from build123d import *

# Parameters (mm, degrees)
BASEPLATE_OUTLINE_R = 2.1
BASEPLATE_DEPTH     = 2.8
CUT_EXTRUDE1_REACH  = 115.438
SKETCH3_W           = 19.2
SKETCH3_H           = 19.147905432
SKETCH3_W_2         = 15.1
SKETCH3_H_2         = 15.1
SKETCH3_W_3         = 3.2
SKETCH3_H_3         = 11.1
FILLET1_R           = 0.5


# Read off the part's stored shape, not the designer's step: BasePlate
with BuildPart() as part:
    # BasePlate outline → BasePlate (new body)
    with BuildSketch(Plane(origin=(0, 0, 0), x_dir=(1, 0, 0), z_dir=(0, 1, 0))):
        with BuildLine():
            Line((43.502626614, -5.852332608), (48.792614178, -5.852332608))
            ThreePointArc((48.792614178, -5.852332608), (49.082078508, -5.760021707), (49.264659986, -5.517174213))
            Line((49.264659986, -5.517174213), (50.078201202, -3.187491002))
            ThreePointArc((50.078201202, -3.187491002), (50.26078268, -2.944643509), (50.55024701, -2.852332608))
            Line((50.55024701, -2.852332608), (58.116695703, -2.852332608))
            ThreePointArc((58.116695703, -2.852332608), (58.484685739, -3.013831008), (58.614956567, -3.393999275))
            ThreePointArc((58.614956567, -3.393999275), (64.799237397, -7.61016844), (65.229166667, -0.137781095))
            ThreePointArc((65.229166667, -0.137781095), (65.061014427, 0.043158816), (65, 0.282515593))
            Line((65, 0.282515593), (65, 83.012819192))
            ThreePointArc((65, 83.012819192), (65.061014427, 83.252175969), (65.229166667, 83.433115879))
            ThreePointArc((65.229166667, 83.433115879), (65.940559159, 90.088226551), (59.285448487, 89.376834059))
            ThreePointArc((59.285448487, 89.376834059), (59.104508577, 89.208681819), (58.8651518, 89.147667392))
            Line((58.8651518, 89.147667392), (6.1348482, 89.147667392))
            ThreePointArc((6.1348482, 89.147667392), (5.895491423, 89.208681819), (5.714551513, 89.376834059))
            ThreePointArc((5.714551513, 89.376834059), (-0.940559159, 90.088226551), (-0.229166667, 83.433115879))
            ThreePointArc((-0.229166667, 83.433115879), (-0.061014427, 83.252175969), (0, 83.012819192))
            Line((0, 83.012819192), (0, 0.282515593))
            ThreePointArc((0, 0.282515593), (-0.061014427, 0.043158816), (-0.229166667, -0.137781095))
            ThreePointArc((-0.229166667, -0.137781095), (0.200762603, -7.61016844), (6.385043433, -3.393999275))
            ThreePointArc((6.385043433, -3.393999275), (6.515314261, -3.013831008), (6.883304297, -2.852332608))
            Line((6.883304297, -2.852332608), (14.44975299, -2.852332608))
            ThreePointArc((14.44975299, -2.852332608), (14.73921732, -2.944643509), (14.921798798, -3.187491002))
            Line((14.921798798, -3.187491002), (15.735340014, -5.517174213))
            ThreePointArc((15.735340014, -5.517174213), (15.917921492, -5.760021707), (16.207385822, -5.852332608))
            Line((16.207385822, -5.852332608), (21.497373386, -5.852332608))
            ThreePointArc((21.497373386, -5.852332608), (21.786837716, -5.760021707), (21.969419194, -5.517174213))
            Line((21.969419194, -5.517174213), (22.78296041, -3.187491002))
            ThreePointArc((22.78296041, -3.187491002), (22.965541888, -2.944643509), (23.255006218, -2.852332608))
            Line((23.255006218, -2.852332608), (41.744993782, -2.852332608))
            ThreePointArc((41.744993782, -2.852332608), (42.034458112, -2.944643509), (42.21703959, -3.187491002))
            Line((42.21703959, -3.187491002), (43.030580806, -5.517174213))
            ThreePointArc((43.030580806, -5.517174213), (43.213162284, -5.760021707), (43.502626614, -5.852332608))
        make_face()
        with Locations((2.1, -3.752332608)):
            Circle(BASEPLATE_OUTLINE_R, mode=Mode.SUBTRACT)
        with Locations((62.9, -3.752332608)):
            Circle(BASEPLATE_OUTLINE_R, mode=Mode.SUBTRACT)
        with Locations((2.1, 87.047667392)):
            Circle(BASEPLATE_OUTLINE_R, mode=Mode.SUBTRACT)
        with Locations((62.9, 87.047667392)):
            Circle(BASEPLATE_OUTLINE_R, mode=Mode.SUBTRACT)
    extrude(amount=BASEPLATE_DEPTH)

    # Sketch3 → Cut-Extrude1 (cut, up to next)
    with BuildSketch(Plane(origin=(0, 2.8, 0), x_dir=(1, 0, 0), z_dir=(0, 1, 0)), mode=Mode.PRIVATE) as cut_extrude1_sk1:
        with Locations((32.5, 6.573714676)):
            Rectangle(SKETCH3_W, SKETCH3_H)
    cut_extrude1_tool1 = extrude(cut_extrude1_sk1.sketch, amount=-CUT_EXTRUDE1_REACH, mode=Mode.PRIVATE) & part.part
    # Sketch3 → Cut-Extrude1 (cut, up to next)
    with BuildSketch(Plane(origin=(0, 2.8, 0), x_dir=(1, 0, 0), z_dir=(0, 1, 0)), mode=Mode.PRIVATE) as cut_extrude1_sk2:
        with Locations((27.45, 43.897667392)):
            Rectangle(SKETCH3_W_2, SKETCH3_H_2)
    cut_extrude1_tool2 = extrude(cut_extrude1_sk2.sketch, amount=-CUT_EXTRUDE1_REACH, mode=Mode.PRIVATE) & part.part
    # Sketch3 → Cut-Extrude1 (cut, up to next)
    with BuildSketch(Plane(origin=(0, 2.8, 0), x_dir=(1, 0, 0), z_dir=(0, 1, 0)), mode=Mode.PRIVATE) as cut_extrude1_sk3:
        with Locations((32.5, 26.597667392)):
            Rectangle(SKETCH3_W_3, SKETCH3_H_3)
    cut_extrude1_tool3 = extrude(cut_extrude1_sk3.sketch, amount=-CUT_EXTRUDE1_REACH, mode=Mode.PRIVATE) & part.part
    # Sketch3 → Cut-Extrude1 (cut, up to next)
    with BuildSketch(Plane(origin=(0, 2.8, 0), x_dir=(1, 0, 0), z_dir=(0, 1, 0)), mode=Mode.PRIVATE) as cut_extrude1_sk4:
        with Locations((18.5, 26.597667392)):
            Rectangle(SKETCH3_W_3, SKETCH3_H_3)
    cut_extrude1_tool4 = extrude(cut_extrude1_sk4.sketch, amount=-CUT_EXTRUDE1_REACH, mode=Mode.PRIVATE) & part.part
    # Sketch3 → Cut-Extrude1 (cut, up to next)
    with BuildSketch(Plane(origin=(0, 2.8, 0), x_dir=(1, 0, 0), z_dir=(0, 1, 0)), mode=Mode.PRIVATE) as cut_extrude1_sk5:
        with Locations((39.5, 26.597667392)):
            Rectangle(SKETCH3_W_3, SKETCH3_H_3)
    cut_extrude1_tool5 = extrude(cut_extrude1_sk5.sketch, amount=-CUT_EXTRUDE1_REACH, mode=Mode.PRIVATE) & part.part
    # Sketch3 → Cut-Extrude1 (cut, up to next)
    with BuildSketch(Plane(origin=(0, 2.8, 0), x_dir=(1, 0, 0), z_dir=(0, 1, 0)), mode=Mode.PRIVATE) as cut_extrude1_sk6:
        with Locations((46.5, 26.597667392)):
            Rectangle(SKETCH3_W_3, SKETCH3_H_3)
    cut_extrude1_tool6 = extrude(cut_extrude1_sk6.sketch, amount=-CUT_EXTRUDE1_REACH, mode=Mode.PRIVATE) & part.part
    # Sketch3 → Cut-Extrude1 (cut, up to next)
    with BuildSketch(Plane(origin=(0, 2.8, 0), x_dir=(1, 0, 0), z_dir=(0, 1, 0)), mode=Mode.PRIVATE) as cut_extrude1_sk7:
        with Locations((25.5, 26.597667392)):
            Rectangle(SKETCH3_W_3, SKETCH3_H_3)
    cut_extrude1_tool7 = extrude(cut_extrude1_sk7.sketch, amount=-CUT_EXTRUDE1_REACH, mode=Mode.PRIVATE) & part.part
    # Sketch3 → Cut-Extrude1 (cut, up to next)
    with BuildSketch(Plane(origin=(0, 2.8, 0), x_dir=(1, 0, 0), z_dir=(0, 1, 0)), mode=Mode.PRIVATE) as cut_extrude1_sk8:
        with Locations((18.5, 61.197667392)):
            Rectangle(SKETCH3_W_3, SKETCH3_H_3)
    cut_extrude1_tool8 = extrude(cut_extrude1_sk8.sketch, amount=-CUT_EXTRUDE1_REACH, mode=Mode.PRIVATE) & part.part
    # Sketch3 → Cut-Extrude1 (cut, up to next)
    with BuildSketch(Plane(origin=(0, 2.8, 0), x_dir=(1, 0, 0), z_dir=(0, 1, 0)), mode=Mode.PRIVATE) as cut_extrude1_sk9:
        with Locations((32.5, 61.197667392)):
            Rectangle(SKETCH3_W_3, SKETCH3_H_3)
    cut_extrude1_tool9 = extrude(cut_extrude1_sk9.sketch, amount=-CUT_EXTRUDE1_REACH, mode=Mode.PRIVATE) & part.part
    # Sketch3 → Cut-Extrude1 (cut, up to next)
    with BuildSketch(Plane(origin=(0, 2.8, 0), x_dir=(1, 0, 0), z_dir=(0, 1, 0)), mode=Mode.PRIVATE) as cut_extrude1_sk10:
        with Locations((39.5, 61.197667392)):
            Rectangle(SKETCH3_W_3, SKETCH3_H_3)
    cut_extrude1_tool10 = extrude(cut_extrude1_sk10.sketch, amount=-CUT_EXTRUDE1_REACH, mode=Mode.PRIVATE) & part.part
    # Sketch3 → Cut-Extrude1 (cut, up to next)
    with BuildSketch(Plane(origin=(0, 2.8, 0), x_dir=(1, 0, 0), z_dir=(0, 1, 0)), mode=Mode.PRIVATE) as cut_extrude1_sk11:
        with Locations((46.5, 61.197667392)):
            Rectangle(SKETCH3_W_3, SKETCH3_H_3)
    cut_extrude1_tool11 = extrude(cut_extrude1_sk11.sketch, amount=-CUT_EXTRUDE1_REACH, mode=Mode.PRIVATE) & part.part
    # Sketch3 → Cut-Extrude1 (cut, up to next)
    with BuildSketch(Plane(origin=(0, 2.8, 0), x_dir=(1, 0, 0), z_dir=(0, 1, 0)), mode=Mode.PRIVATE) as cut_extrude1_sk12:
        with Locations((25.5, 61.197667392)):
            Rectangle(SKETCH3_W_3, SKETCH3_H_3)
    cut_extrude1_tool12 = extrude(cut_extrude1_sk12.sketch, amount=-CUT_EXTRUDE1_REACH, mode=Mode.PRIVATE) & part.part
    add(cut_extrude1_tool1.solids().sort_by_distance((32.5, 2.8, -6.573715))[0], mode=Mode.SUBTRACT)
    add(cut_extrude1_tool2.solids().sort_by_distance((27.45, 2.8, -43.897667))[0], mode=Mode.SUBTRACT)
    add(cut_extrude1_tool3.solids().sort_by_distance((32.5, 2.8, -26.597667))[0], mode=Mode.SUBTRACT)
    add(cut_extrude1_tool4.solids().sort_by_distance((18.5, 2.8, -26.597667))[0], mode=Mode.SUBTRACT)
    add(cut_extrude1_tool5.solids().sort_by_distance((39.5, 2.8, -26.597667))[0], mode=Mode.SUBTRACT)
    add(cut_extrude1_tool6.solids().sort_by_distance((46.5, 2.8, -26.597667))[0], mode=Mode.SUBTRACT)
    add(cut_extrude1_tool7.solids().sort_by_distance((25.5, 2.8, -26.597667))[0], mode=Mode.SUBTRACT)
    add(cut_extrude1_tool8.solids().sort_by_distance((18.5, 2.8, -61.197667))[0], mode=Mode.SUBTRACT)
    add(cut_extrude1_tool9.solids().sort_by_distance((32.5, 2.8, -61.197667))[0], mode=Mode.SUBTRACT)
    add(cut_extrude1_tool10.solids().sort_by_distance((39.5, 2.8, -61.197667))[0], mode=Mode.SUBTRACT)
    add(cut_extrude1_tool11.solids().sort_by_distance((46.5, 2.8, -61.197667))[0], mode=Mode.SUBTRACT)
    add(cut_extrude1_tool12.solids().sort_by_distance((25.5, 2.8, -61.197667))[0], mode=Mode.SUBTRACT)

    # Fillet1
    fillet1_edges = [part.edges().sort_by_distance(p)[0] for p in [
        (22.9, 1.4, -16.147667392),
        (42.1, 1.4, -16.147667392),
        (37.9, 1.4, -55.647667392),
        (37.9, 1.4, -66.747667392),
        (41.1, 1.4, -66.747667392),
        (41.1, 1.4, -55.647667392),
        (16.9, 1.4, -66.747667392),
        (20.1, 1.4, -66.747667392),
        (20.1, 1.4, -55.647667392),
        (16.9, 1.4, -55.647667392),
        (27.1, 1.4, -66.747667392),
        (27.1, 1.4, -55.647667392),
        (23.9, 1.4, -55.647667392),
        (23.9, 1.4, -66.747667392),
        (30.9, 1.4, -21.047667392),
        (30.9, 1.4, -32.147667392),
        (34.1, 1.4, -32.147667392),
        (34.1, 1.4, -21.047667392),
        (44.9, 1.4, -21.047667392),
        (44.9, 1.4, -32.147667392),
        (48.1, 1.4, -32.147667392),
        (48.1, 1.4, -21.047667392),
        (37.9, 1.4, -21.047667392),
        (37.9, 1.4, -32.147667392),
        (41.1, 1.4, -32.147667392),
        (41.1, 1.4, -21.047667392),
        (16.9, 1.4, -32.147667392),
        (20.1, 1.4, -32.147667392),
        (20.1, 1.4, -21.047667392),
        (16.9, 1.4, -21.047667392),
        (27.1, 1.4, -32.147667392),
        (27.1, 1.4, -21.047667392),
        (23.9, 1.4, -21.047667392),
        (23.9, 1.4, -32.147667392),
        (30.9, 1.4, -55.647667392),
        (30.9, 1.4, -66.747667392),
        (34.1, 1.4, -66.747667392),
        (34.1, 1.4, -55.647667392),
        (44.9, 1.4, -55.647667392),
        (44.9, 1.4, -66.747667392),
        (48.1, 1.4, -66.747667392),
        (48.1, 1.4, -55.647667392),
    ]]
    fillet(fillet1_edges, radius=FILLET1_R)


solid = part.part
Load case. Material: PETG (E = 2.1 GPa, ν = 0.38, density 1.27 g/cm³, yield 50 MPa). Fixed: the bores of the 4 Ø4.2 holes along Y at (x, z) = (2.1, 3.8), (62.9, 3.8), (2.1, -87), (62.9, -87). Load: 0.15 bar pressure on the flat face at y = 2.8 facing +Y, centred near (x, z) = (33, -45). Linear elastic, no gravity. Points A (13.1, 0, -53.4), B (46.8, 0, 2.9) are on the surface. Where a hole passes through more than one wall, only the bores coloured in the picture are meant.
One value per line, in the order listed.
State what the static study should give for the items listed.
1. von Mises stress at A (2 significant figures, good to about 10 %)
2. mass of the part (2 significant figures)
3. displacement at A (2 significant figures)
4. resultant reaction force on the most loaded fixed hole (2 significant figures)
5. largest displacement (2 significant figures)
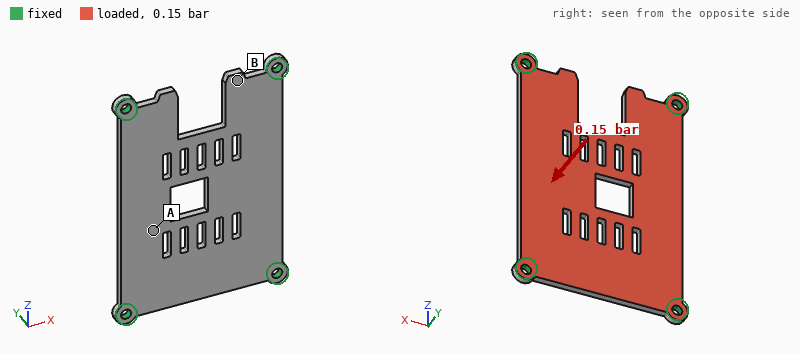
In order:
4.1 MPa
18 g
1.0 mm
21 N
1.4 mm
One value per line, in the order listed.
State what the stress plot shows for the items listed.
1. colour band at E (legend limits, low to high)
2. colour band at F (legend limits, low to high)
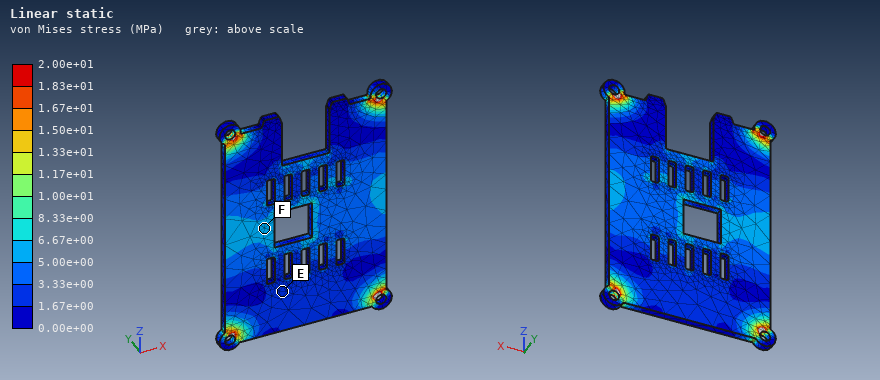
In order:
1.67e+00 to 3.33e+00 MPa
5.00e+00 to 6.67e+00 MPa
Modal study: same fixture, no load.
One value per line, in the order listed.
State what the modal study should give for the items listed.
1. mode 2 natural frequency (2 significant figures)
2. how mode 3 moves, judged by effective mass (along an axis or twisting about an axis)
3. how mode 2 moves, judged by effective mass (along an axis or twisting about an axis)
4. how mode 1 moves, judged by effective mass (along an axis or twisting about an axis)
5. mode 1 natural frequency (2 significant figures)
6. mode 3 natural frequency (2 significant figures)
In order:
550 Hz
twisting about X
twisting about Z
along Y
340 Hz
840 Hz
